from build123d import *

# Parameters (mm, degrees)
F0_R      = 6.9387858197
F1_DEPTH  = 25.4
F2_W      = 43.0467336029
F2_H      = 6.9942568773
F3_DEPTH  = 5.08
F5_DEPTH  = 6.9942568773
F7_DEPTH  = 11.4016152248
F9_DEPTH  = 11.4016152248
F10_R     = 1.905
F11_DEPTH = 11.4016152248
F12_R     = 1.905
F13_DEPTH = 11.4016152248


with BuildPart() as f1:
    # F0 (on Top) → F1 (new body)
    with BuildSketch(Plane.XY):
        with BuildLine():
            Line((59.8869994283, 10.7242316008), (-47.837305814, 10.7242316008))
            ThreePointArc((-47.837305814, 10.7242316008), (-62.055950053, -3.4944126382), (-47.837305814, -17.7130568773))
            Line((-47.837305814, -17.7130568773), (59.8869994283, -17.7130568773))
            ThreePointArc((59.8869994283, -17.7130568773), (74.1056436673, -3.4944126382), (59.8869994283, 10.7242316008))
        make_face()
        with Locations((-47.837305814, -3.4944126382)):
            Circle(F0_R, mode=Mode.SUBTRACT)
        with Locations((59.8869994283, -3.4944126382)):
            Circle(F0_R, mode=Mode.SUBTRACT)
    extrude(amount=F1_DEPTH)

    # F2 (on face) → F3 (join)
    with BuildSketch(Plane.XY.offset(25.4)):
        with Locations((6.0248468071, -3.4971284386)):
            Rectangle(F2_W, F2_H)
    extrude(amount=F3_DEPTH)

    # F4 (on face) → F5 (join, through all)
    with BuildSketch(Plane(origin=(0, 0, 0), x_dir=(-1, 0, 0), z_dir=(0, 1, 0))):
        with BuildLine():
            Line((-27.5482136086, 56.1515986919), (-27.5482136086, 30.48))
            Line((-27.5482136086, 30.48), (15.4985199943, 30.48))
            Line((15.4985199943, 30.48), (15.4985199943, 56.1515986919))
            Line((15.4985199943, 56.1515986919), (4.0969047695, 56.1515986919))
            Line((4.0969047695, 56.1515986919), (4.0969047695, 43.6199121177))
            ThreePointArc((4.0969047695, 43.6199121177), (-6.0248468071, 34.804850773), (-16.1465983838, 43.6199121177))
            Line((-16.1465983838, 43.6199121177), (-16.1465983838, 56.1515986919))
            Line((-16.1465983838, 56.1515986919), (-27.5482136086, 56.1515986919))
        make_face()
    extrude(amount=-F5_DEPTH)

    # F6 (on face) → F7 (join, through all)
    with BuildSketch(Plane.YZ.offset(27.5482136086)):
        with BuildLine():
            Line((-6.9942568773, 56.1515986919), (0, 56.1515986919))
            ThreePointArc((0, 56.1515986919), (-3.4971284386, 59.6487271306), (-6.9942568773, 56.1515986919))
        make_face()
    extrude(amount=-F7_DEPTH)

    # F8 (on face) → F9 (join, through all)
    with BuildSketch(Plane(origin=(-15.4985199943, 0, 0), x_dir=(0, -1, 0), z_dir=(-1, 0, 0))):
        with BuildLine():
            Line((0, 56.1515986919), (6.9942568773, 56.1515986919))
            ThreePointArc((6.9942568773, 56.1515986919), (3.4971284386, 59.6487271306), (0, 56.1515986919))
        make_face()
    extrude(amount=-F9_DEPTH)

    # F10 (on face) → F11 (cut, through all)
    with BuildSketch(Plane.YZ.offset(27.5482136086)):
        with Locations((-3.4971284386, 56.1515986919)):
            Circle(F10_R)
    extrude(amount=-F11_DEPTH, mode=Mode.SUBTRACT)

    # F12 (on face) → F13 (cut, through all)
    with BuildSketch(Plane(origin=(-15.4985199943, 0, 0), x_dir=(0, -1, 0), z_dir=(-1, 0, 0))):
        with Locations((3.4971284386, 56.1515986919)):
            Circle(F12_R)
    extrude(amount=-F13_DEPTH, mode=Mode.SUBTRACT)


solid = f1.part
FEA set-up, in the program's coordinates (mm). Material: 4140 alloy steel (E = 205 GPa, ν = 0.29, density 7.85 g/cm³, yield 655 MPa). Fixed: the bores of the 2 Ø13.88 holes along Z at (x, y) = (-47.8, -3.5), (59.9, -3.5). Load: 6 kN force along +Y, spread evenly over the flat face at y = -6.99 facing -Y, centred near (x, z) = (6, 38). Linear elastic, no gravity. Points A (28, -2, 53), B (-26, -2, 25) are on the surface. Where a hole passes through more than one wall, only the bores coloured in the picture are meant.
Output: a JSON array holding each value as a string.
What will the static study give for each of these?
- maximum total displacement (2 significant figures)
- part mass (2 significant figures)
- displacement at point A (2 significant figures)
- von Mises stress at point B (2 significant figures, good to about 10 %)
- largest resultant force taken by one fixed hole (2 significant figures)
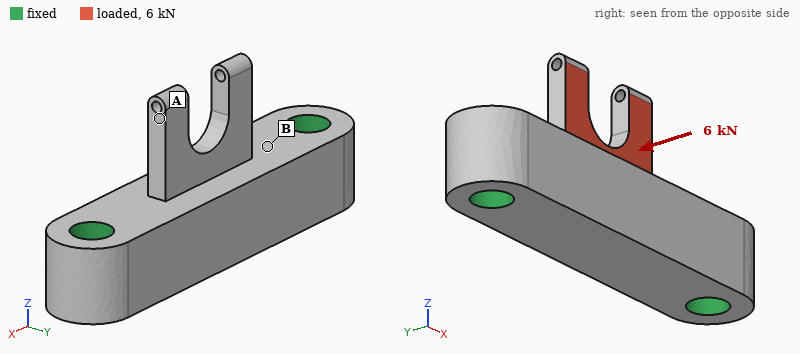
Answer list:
["0.15 mm", "730 g", "0.12 mm", "44 MPa", "3.0 kN"]
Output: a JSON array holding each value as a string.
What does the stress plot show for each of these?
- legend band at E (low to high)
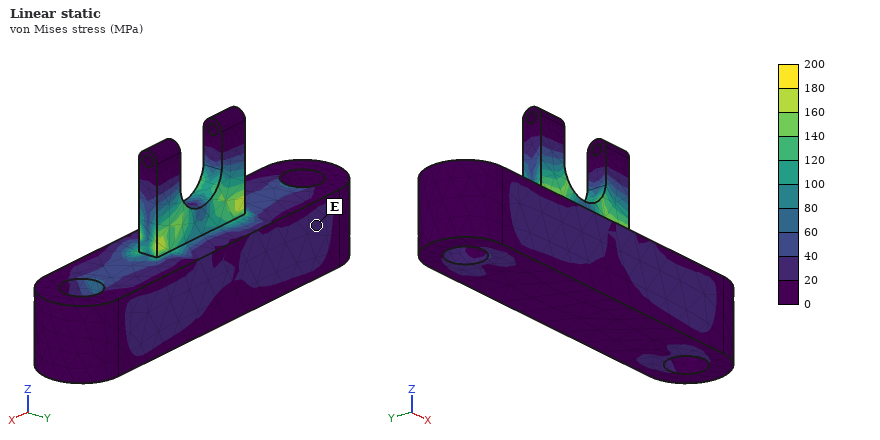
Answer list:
["20 to 40 MPa"]
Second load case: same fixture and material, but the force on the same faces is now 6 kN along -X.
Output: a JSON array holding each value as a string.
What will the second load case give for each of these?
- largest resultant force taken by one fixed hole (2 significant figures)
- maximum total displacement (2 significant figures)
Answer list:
["3.6 kN", "33 µm"]
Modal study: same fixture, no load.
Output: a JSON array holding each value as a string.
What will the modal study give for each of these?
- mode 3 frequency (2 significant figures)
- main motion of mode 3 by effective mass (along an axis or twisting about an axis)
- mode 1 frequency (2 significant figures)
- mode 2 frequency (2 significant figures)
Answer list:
["9300 Hz", "along Y", "5400 Hz", "6100 Hz"]
